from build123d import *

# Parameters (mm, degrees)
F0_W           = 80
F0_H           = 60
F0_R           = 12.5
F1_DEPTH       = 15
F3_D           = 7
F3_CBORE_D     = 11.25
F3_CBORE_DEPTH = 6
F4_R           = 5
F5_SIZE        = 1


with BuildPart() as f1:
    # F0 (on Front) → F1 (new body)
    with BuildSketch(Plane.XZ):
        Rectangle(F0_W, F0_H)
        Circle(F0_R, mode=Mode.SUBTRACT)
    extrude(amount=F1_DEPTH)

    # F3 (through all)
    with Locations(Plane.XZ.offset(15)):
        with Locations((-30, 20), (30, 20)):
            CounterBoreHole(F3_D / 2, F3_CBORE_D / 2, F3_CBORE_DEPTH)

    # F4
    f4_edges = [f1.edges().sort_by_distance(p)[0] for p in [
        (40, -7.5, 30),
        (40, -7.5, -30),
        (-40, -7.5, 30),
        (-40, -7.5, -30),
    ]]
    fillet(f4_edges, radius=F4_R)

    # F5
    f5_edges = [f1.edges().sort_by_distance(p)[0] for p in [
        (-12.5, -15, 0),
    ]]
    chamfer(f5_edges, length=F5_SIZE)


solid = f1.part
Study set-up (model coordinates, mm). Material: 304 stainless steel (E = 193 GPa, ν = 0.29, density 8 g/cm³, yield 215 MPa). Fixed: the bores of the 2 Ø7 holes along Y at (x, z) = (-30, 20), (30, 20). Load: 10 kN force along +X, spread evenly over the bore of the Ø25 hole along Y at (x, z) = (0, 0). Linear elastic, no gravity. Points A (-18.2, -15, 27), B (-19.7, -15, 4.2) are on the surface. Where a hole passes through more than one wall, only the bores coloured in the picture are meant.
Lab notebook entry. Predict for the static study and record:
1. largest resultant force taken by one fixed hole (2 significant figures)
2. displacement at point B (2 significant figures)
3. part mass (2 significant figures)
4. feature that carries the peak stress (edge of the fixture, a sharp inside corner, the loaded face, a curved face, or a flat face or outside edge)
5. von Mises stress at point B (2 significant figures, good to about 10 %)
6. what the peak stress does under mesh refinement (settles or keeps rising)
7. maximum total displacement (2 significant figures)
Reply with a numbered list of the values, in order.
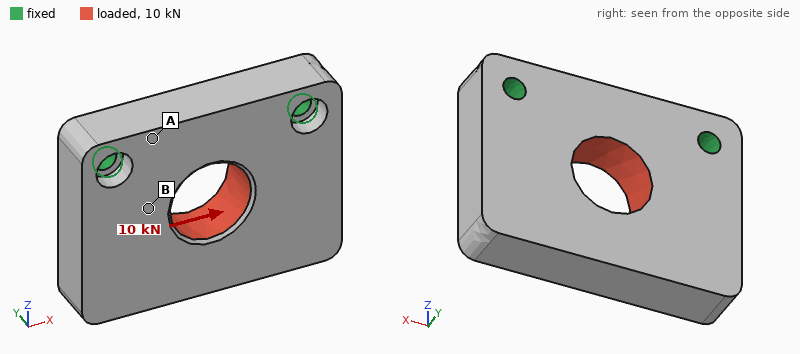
1. 5.8 kN
2. 3.8 µm
3. 500 g
4. edge of the fixture
5. 16 MPa
6. keeps rising
7. 8.8 µm
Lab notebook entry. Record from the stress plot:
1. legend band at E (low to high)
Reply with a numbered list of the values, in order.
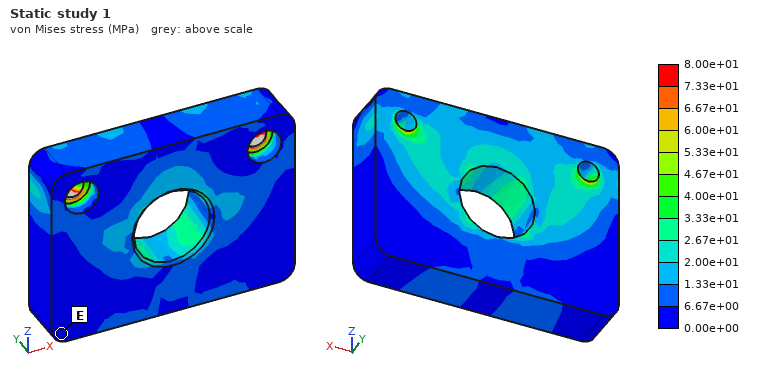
1. 0.00e+00 to 6.67e+00 MPa
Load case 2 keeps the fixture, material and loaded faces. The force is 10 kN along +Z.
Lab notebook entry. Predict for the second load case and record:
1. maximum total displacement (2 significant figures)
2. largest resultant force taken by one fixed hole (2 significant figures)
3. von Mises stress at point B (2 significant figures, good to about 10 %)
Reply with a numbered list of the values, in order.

1. 8.7 µm
2. 5.1 kN
3. 13 MPa
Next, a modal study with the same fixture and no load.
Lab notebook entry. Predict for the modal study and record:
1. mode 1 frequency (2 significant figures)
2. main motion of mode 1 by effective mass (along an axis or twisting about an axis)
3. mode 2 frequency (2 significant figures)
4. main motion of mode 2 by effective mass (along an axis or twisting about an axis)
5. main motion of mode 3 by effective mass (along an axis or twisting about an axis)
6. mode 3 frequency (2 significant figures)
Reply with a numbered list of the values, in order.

1. 2700 Hz
2. along Y
3. 5900 Hz
4. twisting about Z
5. along X
6. 8700 Hz
